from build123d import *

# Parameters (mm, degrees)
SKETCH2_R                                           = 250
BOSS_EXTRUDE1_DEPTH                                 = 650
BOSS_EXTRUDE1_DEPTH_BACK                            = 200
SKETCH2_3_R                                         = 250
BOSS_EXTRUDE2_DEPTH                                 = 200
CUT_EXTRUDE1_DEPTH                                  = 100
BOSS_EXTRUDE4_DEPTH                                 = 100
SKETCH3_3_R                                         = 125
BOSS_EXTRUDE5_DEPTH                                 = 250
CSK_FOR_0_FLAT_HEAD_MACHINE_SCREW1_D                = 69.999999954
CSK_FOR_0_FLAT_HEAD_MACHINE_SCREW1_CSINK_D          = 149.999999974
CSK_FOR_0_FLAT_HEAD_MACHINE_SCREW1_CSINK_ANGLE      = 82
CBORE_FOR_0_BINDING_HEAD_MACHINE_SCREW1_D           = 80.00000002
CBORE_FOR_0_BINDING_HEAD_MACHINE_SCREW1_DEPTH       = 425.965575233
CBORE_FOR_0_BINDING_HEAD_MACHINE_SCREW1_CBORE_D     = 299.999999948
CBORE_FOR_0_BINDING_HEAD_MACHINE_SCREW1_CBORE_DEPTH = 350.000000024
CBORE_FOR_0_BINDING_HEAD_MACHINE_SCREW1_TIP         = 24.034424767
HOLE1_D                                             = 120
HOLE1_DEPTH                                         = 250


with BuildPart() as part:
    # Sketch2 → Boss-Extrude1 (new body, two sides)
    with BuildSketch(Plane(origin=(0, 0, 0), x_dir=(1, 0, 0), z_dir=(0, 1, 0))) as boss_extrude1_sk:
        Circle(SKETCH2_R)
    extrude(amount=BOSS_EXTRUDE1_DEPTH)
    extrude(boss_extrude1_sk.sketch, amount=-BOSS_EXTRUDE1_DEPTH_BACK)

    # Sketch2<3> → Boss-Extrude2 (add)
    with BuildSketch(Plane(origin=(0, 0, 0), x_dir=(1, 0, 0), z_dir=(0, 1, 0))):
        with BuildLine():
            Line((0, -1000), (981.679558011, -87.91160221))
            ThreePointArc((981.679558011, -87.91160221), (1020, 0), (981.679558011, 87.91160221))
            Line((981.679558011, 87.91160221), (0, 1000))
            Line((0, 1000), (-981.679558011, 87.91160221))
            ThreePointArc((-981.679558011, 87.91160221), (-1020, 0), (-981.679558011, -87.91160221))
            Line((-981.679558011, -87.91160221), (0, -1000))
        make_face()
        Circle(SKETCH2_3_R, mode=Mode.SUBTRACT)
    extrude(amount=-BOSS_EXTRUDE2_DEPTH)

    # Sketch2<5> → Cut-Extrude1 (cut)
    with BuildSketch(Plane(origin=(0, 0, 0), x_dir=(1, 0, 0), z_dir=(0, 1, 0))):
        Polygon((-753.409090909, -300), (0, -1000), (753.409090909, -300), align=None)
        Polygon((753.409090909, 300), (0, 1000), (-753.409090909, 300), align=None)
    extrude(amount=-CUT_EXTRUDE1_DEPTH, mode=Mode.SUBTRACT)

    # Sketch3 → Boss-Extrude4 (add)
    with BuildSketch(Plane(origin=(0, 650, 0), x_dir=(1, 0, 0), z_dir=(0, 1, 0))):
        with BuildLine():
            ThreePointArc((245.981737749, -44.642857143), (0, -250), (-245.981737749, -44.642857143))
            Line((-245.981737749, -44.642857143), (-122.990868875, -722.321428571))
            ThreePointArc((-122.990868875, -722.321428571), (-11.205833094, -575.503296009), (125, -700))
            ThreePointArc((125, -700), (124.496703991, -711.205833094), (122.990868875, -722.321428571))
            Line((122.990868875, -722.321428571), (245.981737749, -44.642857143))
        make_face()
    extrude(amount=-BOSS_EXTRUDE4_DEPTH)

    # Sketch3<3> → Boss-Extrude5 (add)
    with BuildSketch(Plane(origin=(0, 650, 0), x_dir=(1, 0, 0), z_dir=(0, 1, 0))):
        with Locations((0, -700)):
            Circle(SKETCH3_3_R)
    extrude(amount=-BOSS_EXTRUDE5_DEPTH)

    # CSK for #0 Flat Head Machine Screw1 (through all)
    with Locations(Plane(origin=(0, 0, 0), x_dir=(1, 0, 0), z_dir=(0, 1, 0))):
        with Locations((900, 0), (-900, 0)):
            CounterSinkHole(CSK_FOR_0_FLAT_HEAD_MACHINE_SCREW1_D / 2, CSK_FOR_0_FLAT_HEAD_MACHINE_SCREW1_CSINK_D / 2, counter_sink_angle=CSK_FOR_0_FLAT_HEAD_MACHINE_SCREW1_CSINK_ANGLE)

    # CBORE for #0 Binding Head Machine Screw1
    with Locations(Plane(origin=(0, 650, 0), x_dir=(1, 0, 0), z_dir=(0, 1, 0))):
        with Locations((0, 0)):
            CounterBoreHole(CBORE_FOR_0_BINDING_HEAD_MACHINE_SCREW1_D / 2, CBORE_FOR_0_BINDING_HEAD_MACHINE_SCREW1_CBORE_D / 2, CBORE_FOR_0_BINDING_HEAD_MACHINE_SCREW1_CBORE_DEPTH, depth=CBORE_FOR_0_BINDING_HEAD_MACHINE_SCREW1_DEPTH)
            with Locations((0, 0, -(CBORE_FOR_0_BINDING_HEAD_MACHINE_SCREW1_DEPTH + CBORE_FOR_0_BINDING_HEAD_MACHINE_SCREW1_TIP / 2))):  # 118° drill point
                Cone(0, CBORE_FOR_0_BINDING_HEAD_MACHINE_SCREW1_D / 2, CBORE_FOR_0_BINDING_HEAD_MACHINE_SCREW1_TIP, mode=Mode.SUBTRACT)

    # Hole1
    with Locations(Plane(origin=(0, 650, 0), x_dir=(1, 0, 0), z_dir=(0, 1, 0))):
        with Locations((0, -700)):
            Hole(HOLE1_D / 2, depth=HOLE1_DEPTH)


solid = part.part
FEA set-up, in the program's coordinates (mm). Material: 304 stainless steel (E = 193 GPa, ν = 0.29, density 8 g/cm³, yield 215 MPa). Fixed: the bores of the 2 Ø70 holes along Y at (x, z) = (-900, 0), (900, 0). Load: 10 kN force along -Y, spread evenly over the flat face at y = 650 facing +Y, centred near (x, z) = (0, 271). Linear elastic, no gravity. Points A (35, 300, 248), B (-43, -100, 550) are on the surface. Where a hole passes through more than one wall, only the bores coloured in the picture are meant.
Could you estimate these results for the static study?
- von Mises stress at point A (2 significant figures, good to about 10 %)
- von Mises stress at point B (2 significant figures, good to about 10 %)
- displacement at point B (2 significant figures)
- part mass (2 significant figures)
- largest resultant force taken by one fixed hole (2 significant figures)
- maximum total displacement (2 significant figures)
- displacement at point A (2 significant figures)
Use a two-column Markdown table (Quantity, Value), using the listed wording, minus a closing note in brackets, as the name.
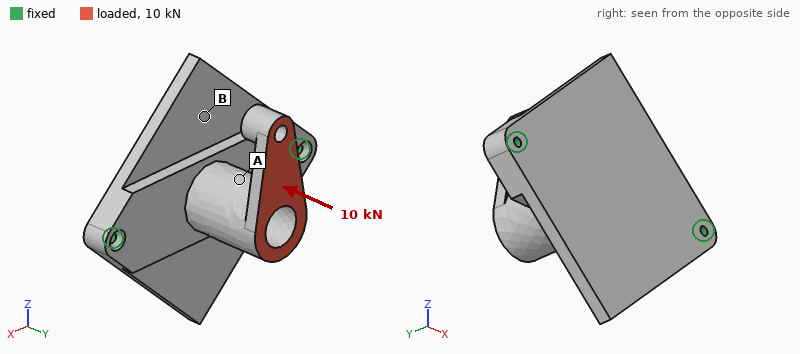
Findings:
| Quantity | Value |
|---|---|
| von Mises stress at point A | 0.30 MPa |
| von Mises stress at point B | 0.15 MPa |
| displacement at point B | 11 µm |
| part mass | 3600 kg |
| largest resultant force taken by one fixed hole | 5.1 kN |
| maximum total displacement | 47 µm |
| displacement at point A | 9.8 µm |
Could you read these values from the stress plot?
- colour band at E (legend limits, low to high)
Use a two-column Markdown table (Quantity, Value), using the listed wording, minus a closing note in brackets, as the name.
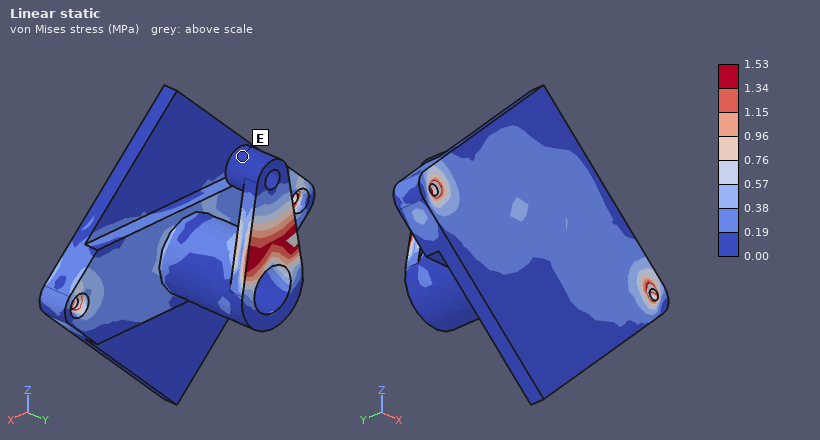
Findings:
| Quantity | Value |
|---|---|
| colour band at E | 0.00 to 0.19 MPa |
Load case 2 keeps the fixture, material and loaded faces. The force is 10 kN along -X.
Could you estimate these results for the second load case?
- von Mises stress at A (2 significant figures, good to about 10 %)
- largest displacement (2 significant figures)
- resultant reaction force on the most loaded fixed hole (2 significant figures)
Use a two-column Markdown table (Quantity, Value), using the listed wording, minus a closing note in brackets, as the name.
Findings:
| Quantity | Value |
|---|---|
| von Mises stress at A | 0.40 MPa |
| largest displacement | 15 µm |
| resultant reaction force on the most loaded fixed hole | 7.3 kN |
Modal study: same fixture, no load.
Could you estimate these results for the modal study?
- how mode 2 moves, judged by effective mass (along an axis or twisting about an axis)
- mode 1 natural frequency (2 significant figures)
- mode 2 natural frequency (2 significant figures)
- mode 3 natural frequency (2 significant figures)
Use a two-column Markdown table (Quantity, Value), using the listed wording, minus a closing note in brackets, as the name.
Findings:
| Quantity | Value |
|---|---|
| how mode 2 moves, judged by effective mass | along Y |
| mode 1 natural frequency | 91 Hz |
| mode 2 natural frequency | 140 Hz |
| mode 3 natural frequency | 180 Hz |
